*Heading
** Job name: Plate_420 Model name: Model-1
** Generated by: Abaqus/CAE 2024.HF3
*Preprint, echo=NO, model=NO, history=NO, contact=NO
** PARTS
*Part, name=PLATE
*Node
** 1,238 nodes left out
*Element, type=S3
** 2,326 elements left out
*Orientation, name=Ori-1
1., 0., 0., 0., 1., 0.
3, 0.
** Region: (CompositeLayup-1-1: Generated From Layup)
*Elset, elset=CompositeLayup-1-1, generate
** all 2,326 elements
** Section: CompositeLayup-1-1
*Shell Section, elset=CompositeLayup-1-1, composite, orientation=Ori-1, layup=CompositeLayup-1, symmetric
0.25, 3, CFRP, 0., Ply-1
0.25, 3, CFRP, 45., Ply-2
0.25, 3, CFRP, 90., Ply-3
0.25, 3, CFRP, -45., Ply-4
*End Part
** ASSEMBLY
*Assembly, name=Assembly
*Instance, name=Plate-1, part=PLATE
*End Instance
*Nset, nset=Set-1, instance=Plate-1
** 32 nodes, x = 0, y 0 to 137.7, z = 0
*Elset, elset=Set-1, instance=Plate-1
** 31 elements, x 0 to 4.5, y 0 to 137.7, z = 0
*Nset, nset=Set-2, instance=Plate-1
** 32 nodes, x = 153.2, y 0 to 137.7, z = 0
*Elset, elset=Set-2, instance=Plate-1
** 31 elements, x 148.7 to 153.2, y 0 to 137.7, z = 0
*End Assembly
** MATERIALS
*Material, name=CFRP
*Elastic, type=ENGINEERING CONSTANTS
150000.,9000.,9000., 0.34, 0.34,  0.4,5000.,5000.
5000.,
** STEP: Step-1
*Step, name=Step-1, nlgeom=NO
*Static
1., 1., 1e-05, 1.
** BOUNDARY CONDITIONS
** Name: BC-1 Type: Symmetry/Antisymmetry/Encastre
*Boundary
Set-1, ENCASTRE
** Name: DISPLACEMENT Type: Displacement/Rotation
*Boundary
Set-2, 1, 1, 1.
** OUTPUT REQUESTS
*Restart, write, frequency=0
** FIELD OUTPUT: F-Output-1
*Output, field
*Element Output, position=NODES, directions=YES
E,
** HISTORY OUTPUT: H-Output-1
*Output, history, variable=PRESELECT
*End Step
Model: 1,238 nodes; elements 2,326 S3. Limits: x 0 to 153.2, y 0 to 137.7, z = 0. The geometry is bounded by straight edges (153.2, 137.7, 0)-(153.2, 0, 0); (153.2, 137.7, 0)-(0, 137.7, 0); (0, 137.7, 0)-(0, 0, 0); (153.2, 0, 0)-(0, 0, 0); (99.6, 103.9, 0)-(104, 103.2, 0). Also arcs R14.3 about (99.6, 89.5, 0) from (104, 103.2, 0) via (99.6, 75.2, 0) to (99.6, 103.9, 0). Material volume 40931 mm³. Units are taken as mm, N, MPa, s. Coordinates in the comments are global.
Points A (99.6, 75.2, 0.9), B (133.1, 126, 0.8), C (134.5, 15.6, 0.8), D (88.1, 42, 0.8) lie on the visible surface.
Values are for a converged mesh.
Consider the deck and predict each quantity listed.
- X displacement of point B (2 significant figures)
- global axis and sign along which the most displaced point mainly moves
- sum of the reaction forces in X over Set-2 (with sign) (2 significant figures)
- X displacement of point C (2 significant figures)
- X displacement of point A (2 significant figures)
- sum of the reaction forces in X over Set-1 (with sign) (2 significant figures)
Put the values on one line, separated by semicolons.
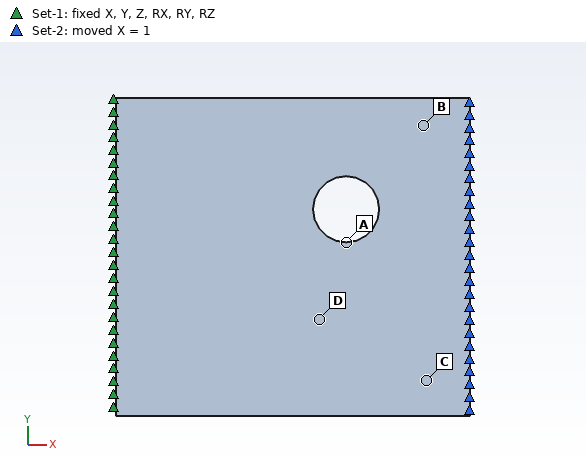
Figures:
0.86 mm; +X; 95000 N; 0.87 mm; 0.62 mm; -95000 N
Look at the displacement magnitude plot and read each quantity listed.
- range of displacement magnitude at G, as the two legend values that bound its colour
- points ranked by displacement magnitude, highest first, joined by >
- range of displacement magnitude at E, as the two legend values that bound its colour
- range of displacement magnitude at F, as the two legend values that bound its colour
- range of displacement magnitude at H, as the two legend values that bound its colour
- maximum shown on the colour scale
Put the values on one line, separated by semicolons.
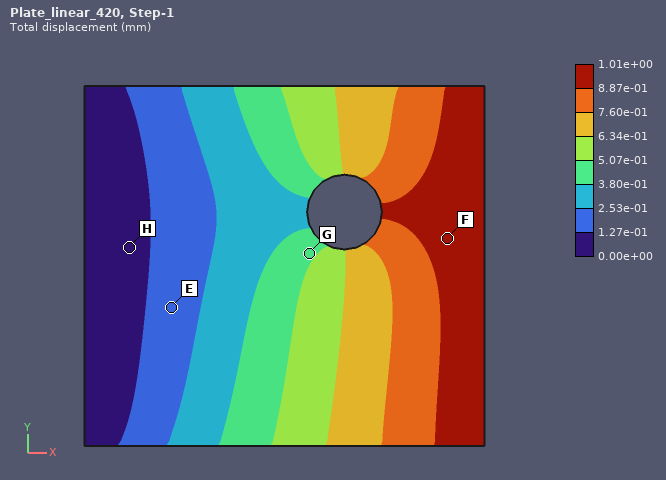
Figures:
3.80e-01 to 5.07e-01 mm; F > G > E > H; 1.27e-01 to 2.53e-01 mm; 8.87e-01 to 1.01e+00 mm; 0.00e+00 to 1.27e-01 mm; 1.01e+00 mm
